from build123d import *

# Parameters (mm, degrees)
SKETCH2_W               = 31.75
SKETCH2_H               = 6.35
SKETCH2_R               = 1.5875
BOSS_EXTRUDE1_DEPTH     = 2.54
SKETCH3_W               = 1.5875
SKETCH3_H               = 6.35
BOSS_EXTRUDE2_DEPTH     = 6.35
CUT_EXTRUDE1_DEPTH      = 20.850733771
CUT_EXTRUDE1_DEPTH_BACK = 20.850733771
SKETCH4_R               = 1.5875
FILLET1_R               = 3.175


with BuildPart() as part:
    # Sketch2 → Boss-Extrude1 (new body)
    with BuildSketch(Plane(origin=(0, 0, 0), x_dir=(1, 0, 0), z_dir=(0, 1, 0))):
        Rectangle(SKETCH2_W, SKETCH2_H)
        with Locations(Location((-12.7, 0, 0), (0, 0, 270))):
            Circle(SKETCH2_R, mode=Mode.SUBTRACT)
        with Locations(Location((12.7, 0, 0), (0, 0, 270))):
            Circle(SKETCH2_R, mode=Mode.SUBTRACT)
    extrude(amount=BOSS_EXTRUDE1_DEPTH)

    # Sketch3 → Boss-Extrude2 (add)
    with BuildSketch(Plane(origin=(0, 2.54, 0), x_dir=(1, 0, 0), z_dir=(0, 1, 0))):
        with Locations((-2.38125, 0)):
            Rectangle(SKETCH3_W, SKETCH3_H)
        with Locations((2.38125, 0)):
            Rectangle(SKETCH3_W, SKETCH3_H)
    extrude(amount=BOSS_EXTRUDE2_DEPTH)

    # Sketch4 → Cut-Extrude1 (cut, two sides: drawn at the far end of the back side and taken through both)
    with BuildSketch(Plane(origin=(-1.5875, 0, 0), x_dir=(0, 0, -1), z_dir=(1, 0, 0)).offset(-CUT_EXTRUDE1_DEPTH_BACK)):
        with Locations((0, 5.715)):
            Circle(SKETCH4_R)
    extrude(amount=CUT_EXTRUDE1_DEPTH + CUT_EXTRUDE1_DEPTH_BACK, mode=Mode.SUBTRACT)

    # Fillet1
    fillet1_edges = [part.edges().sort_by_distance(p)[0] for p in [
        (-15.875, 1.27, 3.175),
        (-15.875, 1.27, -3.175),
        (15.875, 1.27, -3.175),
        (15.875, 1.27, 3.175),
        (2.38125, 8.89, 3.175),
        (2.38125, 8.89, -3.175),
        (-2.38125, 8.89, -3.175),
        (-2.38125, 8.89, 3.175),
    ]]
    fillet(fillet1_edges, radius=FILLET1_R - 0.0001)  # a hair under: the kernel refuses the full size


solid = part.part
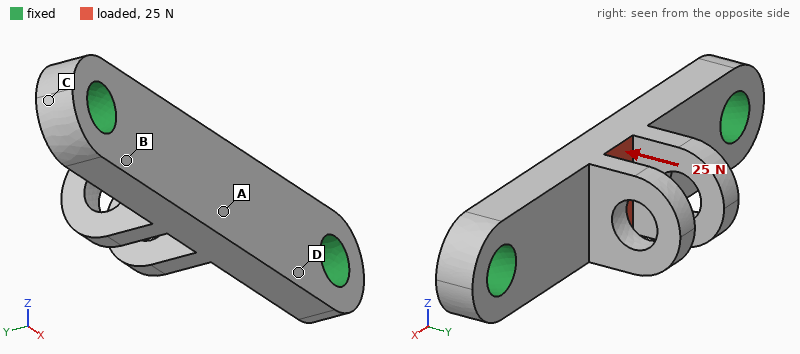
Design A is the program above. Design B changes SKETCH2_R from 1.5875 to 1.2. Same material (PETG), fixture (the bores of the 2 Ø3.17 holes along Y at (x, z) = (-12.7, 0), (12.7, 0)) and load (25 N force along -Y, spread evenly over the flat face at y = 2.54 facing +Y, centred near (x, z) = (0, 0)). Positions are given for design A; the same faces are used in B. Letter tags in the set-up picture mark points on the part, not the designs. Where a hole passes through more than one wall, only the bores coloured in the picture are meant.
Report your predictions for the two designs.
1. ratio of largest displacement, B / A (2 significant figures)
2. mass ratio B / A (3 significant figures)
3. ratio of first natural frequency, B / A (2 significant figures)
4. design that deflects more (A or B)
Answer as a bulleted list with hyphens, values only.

- 1.1
- 1.03
- 0.93
- B
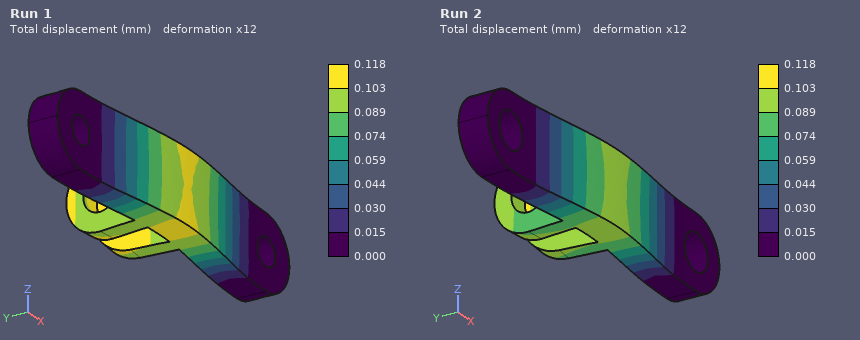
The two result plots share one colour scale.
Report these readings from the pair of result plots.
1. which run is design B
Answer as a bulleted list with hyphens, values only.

- Run 1
